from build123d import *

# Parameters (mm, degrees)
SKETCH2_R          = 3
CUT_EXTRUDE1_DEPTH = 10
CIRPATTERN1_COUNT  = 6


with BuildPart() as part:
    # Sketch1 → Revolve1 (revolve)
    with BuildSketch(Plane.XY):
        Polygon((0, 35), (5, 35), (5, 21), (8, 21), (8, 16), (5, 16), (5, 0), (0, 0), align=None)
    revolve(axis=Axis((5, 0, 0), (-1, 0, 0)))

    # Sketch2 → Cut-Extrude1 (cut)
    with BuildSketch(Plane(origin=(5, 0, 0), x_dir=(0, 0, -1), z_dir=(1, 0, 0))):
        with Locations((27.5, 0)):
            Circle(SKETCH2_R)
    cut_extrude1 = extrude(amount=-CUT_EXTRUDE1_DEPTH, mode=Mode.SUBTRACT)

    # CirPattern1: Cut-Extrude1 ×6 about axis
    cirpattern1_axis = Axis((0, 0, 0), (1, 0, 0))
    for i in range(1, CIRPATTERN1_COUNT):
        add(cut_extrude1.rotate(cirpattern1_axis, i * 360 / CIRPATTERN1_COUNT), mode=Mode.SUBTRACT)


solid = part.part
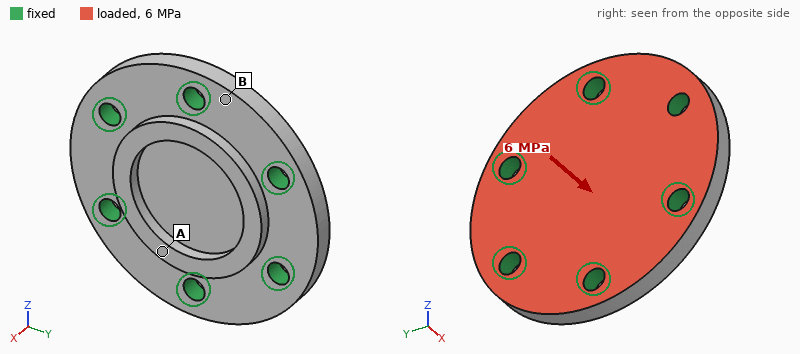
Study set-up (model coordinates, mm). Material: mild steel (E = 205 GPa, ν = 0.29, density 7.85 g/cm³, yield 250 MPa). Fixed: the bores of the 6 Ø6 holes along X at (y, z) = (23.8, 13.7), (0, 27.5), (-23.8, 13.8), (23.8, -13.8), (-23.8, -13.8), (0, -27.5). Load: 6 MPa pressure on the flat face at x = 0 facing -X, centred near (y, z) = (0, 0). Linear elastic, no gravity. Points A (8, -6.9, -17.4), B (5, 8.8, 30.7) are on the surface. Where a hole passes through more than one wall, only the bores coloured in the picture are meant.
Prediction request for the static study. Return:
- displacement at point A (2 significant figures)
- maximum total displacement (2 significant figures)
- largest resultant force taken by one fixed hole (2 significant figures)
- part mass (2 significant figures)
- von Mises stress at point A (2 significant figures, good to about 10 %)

8.7 µm
21 µm
3.7 kN
160 g
64 MPa
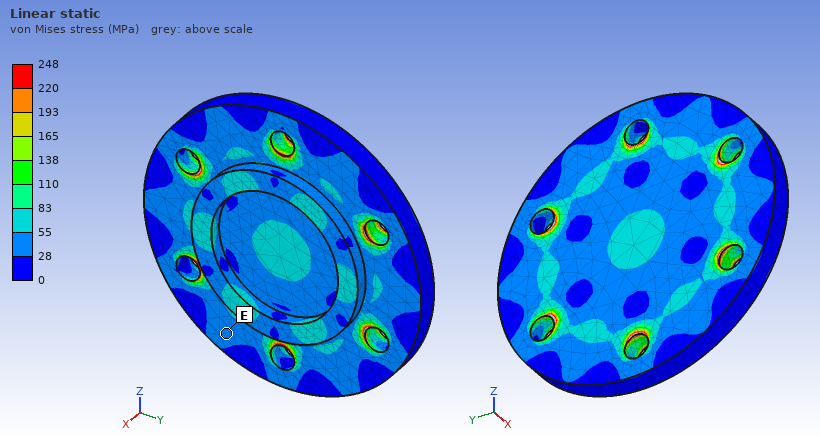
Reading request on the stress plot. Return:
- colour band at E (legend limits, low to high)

28 to 55 MPa
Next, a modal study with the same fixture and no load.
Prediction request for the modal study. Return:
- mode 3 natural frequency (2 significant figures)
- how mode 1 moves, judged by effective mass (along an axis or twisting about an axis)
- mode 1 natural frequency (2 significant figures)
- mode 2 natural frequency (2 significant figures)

28 kHz
along X
16 kHz
28 kHz
